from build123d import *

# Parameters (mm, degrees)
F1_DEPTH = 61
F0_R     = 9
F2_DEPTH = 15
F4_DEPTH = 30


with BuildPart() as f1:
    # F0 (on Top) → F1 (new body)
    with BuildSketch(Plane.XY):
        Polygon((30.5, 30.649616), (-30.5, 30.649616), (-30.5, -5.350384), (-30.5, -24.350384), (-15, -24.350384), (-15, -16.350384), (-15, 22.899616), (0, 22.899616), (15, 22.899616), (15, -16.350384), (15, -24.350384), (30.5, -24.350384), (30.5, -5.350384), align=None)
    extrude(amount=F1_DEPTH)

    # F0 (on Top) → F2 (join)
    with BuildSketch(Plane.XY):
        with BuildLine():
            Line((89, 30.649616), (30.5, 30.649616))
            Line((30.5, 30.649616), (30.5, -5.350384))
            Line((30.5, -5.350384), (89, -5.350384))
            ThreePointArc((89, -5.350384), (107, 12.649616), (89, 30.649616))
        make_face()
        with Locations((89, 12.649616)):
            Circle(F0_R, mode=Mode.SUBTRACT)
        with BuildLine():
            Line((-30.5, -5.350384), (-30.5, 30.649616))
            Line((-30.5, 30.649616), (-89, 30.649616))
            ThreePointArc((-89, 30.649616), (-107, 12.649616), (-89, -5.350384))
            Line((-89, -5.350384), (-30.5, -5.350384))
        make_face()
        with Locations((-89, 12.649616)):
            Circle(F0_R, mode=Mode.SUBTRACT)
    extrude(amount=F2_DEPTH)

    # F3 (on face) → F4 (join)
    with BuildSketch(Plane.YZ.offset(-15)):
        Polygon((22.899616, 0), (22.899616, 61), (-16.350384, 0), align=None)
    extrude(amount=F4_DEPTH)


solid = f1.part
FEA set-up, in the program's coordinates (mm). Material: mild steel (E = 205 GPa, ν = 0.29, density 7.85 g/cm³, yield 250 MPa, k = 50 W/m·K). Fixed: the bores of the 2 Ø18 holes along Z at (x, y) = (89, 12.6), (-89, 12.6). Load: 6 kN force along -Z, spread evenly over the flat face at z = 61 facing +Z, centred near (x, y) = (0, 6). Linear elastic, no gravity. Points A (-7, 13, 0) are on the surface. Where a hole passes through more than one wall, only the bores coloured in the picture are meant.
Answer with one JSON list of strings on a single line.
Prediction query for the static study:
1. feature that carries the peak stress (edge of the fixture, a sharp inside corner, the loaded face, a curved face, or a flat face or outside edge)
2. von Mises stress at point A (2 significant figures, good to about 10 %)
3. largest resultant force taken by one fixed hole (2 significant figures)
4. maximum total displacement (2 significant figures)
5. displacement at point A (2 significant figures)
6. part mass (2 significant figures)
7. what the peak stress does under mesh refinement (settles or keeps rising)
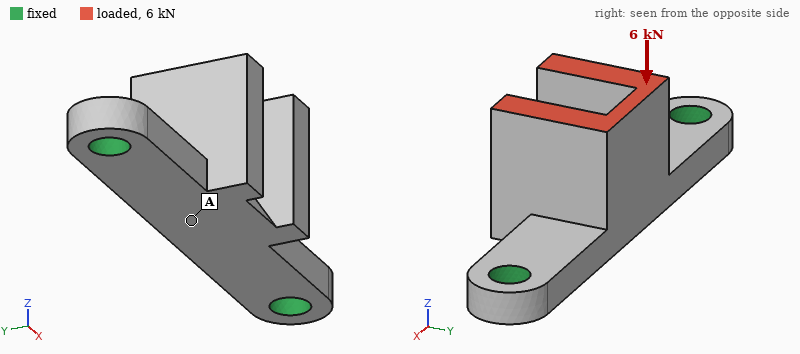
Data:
["edge of the fixture", "13 MPa", "3.3 kN", "52 µm", "31 µm", "1.8 kg", "keeps rising"]
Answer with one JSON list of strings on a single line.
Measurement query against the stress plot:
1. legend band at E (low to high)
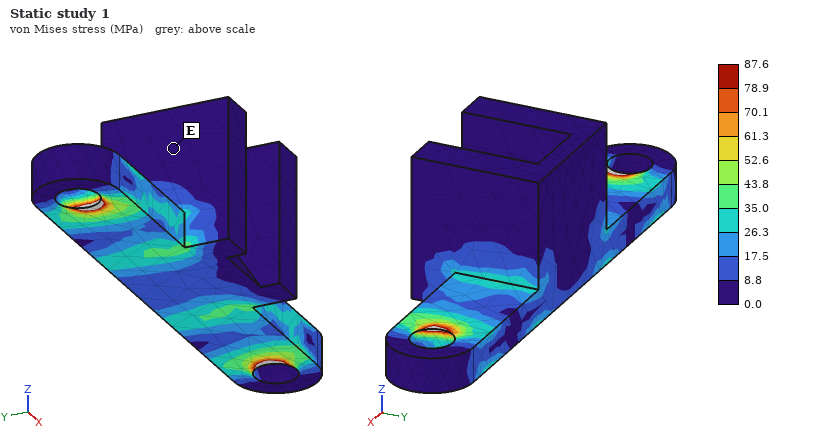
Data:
["0.0 to 8.8 MPa"]
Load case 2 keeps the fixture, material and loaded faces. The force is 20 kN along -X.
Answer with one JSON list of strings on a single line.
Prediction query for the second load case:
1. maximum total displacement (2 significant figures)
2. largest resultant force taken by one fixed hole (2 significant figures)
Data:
["0.15 mm", "13 kN"]
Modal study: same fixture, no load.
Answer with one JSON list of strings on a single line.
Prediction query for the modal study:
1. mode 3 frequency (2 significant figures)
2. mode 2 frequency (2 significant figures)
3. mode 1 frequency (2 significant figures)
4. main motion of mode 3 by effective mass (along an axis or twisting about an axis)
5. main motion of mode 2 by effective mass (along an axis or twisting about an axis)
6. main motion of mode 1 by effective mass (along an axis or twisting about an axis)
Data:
["3200 Hz", "1900 Hz", "1300 Hz", "along X", "along Z", "along Y"]
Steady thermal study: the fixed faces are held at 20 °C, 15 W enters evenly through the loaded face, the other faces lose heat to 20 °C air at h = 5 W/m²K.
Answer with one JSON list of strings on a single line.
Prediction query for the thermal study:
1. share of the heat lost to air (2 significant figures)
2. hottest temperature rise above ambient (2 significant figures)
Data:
["13 %", "21 K"]
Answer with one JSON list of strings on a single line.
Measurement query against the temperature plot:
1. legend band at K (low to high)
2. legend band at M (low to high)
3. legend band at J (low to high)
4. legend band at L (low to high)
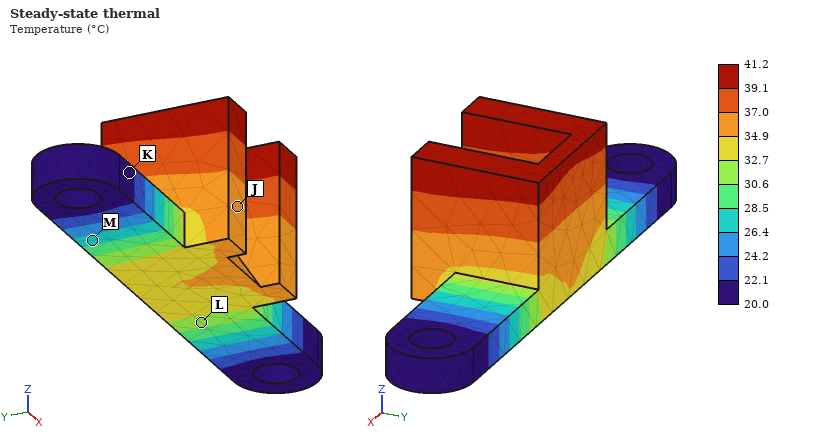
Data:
["20.0 to 22.1 °C", "26.4 to 28.5 °C", "34.9 to 37.0 °C", "30.6 to 32.7 °C"]
